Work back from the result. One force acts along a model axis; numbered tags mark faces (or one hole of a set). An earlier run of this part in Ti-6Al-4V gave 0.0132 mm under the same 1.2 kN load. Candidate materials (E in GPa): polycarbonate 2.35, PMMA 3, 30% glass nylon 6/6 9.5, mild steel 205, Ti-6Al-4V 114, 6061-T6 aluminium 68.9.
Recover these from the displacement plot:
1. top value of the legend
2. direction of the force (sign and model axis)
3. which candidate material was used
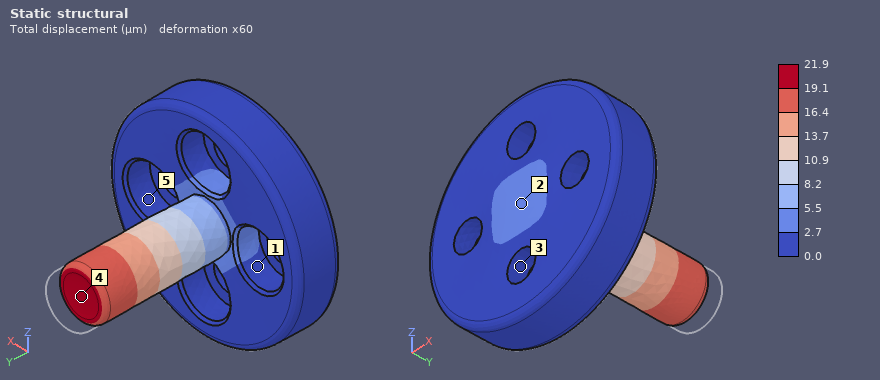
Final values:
21.9 µm
-Y
6061-T6 aluminium
